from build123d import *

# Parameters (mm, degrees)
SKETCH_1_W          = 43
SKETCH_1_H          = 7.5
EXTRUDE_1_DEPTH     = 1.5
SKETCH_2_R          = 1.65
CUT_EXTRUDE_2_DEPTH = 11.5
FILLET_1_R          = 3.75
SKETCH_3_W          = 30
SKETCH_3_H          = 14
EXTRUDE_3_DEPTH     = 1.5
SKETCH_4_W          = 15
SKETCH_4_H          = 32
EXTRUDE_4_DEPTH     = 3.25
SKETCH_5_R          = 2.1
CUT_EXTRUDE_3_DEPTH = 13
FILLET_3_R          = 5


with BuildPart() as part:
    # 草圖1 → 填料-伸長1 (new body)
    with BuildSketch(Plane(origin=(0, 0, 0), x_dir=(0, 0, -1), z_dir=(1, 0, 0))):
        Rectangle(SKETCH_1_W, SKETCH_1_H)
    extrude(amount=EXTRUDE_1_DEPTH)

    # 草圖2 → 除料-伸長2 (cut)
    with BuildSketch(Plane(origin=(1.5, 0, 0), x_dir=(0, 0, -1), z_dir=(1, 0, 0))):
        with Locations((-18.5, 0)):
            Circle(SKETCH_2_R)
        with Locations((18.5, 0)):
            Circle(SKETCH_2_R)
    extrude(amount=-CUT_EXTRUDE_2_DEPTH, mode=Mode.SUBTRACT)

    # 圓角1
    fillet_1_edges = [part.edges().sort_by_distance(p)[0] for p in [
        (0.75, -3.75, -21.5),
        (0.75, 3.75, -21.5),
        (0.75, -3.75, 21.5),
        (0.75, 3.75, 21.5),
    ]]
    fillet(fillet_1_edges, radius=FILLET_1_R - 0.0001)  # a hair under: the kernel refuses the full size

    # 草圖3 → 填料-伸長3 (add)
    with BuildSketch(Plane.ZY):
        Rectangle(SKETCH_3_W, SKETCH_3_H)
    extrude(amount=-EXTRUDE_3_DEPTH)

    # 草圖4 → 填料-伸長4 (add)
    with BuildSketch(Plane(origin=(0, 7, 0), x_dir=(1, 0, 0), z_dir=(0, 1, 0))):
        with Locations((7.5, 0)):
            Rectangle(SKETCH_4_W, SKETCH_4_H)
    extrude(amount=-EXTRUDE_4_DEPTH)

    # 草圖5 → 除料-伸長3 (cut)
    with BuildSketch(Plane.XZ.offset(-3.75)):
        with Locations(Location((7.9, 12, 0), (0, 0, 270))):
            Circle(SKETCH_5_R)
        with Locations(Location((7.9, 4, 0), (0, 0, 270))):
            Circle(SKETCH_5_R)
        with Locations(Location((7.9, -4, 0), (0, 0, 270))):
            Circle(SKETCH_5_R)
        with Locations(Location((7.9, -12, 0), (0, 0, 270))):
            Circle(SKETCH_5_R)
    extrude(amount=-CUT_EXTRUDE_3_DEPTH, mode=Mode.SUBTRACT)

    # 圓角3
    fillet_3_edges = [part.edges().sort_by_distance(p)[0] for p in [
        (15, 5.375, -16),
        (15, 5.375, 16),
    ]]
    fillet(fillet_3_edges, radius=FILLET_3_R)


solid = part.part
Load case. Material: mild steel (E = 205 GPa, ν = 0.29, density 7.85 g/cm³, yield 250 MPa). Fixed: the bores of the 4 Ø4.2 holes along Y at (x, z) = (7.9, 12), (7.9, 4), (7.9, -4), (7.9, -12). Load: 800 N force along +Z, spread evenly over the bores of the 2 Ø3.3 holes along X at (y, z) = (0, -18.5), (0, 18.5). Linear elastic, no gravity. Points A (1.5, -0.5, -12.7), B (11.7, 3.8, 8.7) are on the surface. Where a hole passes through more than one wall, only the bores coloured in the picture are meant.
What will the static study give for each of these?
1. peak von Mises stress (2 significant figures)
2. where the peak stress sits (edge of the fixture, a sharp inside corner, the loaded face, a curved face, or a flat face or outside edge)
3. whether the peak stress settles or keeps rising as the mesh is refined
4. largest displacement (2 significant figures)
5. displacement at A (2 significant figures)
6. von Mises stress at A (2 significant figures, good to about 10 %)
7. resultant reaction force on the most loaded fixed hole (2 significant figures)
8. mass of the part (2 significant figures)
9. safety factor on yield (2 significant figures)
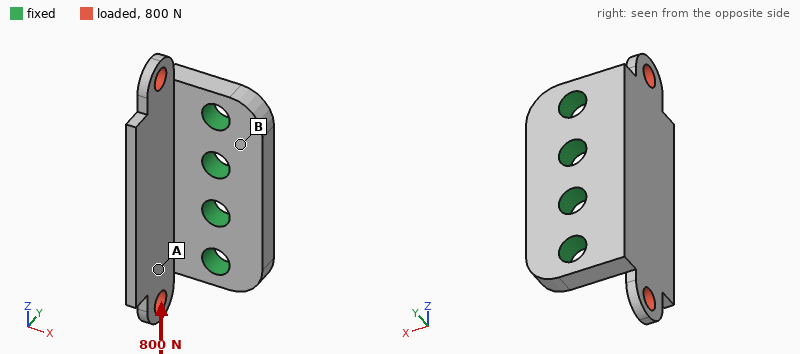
110 MPa
the loaded face
settles
7.3 µm
3.9 µm
28 MPa
290 N
15 g
2.3
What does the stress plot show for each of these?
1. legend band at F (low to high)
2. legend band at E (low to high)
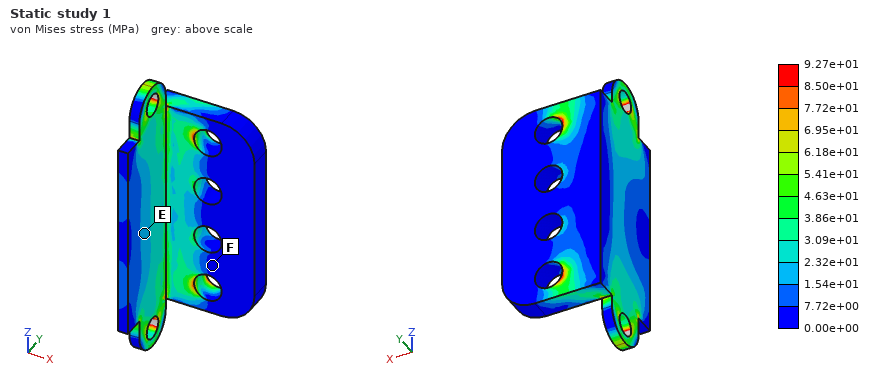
0.00e+00 to 7.72e+00 MPa
1.54e+01 to 2.32e+01 MPa
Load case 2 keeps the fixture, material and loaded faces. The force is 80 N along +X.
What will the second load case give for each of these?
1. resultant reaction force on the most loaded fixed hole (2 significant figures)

60 N
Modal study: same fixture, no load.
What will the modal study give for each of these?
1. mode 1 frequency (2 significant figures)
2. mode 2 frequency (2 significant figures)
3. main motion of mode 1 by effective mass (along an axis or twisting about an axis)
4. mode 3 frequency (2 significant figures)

8800 Hz
11 kHz
along X
16 kHz
